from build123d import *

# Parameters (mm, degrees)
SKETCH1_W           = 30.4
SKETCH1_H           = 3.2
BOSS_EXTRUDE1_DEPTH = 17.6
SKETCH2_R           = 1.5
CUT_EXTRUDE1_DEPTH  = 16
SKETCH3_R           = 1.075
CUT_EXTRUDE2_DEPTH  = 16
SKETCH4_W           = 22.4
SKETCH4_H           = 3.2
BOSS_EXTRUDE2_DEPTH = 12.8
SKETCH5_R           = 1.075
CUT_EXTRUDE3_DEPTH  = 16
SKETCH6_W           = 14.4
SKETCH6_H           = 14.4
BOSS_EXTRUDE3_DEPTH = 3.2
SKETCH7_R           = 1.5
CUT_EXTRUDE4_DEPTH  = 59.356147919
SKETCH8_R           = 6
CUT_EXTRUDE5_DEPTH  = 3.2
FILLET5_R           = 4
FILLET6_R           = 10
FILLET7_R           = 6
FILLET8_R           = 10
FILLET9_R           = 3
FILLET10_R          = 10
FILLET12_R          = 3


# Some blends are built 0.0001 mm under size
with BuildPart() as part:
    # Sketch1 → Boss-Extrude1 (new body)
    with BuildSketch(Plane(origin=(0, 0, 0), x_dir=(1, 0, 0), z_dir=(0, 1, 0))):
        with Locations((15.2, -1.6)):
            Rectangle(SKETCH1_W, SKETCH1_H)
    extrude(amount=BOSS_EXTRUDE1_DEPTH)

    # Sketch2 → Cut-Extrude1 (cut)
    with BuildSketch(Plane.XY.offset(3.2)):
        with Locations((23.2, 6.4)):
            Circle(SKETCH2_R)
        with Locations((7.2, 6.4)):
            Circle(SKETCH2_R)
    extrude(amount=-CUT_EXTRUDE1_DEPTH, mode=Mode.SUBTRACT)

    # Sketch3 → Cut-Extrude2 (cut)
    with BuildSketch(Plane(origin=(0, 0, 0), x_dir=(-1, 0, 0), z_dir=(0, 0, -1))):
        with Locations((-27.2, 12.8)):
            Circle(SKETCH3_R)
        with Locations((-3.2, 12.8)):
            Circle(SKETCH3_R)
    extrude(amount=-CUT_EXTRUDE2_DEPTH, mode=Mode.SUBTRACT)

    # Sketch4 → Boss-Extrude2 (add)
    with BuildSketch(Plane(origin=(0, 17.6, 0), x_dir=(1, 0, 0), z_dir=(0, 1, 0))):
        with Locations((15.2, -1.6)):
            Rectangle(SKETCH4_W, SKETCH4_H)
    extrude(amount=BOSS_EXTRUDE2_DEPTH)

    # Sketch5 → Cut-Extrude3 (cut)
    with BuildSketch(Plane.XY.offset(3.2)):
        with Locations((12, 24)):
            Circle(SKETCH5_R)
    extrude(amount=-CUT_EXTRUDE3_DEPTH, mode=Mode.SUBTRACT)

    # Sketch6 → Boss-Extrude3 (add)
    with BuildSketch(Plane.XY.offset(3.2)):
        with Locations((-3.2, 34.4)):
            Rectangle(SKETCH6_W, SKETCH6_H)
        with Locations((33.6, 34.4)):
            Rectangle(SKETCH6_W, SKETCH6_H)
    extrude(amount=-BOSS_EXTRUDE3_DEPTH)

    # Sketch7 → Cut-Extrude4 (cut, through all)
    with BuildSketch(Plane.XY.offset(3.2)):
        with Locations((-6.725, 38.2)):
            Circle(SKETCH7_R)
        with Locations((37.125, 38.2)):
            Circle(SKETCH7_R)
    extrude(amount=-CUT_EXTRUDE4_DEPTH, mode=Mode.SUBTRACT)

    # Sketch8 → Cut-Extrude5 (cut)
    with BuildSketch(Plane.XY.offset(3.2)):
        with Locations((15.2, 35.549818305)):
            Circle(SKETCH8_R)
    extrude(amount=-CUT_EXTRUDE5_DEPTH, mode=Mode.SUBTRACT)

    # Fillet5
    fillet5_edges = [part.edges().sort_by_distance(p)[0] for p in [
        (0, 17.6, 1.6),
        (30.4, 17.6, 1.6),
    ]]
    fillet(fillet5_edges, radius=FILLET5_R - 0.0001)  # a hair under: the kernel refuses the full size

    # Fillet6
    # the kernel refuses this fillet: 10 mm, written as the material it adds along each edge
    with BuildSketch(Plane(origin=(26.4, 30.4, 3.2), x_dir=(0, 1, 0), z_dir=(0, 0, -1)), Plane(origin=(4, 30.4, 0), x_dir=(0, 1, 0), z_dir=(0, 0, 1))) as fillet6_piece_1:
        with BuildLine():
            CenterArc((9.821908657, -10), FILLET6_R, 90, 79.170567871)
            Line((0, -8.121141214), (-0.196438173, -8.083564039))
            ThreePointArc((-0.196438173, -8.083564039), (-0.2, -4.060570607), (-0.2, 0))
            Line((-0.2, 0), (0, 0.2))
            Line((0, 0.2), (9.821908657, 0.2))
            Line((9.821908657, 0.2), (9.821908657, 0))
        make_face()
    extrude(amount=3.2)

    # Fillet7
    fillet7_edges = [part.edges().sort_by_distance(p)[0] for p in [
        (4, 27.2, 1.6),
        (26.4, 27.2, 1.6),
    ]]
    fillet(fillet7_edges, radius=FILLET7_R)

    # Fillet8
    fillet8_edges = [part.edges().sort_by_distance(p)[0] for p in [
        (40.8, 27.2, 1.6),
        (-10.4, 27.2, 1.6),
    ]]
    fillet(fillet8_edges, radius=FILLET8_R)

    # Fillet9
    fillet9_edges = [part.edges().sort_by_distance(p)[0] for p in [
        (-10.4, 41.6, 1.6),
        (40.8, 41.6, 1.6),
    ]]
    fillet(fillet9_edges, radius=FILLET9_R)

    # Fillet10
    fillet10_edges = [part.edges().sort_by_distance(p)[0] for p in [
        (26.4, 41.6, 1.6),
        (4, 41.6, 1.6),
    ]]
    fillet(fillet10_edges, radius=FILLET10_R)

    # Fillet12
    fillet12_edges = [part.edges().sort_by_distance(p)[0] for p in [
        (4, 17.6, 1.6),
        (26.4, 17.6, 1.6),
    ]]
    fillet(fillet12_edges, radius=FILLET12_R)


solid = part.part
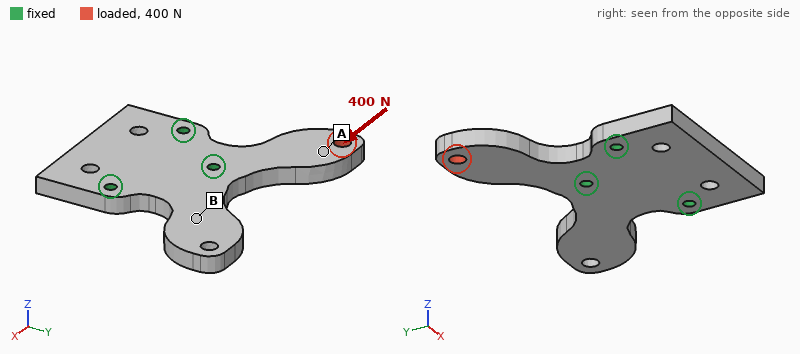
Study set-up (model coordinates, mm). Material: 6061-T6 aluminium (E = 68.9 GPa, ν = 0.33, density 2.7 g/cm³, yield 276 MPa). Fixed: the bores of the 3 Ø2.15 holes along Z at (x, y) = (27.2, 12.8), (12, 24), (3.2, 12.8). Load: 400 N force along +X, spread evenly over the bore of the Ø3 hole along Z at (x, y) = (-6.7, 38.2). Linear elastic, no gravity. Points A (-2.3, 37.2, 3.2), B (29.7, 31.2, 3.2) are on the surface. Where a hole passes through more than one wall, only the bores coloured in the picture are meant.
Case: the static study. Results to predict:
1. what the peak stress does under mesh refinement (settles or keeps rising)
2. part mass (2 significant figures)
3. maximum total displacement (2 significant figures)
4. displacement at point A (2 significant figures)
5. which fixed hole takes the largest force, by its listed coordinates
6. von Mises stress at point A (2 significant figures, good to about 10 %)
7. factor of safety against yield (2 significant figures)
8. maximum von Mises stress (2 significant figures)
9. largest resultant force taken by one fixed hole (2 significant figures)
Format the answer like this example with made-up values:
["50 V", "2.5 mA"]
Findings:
["settles", "10 g", "75 µm", "47 µm", "(12, 24)", "21 MPa", "2.4", "120 MPa", "510 N"]
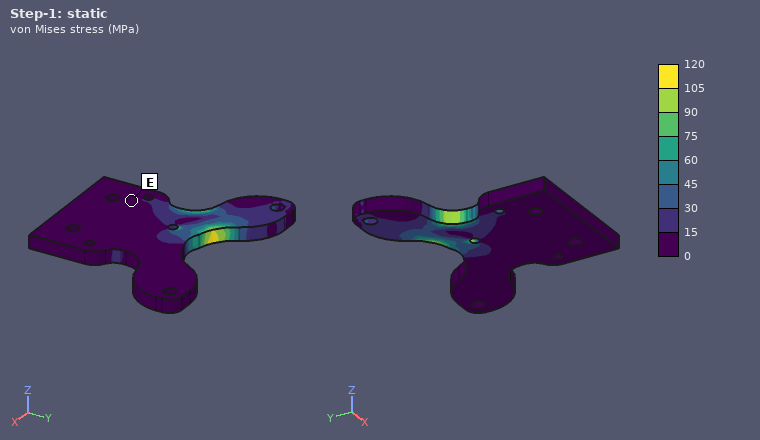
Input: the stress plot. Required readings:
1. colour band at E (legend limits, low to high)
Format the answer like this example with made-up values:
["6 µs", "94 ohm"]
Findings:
["0 to 15 MPa"]
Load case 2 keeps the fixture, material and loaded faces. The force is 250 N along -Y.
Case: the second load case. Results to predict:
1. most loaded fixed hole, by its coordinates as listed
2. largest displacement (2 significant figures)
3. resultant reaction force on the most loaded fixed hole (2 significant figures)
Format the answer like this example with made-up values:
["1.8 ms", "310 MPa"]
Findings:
["(3.2, 12.8)", "58 µm", "250 N"]
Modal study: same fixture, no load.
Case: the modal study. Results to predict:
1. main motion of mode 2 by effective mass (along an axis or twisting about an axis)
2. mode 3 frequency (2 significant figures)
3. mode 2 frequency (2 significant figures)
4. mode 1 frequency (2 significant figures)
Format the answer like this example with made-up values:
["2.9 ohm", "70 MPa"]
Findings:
["along Z", "11 kHz", "4000 Hz", "3200 Hz"]
